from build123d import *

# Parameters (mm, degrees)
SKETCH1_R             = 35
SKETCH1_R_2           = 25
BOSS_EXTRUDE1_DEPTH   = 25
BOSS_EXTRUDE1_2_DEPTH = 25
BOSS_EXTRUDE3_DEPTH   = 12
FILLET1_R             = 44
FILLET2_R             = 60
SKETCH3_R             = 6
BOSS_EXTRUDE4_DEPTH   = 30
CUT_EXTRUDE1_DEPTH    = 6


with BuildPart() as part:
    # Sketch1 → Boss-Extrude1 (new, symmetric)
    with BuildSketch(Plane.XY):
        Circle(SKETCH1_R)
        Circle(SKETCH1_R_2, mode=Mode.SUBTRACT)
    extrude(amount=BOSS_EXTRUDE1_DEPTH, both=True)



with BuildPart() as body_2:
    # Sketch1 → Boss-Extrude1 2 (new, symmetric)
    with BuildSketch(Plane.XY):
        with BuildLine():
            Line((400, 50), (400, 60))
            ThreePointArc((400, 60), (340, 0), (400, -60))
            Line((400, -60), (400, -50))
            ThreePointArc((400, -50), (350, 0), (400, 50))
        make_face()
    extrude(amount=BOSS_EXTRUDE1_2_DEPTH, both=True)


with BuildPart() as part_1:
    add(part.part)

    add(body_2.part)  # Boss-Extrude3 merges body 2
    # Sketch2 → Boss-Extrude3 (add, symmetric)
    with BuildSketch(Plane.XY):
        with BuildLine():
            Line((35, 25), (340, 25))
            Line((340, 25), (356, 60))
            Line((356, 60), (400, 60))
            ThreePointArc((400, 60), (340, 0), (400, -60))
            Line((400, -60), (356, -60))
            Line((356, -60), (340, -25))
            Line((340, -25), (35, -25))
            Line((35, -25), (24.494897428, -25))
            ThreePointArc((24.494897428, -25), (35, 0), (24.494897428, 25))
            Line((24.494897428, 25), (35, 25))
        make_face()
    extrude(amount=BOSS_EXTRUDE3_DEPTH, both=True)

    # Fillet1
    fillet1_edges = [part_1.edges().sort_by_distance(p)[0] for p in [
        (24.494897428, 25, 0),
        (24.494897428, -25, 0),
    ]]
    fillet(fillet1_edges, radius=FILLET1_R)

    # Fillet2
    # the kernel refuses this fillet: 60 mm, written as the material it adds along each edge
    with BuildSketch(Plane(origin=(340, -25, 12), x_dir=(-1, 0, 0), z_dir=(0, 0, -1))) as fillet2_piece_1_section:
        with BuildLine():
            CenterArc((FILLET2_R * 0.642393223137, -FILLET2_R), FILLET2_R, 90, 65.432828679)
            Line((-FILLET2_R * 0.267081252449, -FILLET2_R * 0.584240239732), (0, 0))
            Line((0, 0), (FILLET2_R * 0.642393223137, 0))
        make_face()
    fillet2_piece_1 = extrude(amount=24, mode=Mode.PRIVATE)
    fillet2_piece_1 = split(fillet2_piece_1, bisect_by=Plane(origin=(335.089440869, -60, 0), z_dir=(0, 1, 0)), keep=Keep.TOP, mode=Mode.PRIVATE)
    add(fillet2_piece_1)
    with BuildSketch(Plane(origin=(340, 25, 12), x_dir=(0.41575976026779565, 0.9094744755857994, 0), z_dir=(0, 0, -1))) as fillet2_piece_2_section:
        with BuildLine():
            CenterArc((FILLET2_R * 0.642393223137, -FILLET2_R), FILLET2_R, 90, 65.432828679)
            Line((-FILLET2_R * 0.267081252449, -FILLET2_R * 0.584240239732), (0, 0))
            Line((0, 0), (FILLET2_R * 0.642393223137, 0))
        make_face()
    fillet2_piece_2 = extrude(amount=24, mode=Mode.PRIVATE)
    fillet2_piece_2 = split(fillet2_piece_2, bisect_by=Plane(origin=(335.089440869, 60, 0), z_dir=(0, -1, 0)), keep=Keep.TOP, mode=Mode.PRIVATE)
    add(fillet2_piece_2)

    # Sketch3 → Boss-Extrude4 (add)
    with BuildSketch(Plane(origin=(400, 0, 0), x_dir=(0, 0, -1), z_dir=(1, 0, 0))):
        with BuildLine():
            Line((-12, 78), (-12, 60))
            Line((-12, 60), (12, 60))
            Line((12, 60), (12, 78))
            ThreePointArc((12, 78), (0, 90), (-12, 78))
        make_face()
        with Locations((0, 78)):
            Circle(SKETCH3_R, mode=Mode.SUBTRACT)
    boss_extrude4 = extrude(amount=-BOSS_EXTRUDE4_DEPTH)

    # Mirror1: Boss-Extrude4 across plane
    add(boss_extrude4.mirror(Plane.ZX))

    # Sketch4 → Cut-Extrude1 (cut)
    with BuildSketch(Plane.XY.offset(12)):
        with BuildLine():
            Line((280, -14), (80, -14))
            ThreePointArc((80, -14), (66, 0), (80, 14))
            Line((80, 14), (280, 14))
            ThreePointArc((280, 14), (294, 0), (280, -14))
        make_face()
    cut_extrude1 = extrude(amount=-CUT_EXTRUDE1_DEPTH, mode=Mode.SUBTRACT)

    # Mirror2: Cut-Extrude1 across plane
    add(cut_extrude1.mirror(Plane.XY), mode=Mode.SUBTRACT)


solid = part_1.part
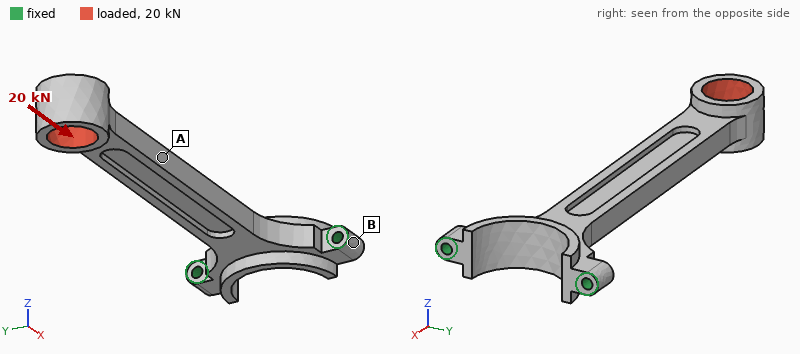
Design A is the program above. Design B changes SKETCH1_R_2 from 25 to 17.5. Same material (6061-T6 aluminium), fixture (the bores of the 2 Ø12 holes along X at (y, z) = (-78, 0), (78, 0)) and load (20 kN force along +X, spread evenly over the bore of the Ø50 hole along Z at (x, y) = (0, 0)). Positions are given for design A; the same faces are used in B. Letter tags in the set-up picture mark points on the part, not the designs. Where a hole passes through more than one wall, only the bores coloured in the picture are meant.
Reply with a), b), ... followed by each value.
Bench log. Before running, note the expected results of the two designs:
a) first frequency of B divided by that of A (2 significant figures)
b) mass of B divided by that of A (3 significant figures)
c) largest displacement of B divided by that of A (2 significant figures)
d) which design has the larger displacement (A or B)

a) 0.87
b) 1.09
c) 0.78
d) A
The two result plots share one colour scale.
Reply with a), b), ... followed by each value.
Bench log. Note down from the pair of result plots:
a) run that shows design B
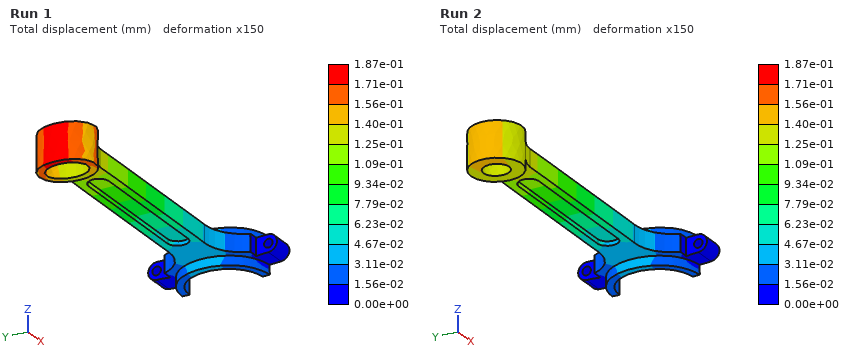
a) Run 2
